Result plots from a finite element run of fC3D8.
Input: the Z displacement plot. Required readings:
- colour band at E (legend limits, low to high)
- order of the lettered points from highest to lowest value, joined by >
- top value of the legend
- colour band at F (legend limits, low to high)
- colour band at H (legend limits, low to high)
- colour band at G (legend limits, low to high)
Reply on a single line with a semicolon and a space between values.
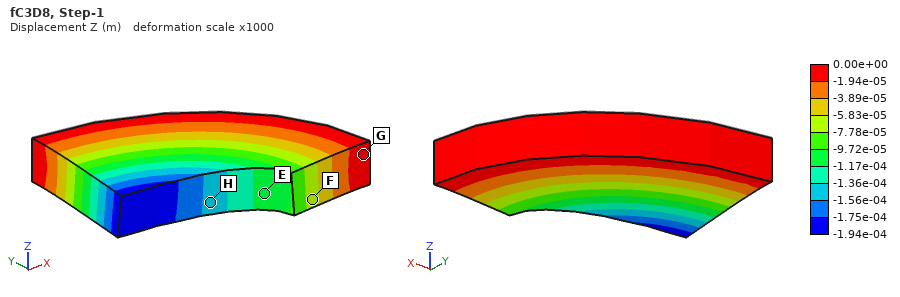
-1.17e-04 to -9.72e-05 m; G > F > E > H; 0.00e+00 m; -7.78e-05 to -5.83e-05 m; -1.56e-04 to -1.36e-04 m; -1.94e-05 to 0.00e+00 m
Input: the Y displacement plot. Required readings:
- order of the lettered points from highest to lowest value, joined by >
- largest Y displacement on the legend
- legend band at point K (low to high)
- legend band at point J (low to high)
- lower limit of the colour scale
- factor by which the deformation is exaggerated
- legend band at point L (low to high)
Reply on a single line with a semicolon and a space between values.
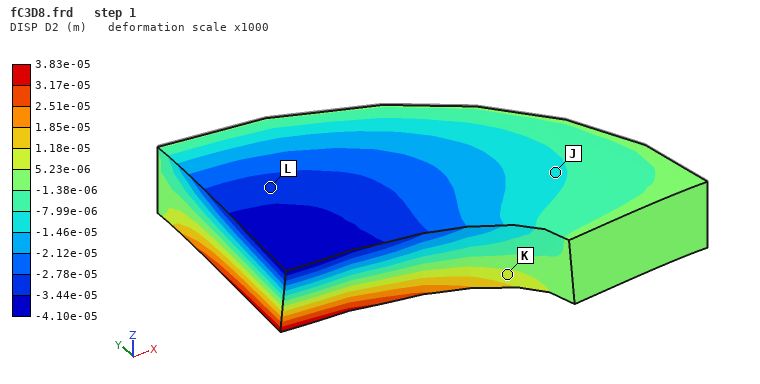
K > J > L; 3.83e-05 m; 5.23e-06 to 1.18e-05 m; -1.46e-05 to -7.99e-06 m; -4.10e-05 m; 1000; -3.44e-05 to -2.78e-05 m
